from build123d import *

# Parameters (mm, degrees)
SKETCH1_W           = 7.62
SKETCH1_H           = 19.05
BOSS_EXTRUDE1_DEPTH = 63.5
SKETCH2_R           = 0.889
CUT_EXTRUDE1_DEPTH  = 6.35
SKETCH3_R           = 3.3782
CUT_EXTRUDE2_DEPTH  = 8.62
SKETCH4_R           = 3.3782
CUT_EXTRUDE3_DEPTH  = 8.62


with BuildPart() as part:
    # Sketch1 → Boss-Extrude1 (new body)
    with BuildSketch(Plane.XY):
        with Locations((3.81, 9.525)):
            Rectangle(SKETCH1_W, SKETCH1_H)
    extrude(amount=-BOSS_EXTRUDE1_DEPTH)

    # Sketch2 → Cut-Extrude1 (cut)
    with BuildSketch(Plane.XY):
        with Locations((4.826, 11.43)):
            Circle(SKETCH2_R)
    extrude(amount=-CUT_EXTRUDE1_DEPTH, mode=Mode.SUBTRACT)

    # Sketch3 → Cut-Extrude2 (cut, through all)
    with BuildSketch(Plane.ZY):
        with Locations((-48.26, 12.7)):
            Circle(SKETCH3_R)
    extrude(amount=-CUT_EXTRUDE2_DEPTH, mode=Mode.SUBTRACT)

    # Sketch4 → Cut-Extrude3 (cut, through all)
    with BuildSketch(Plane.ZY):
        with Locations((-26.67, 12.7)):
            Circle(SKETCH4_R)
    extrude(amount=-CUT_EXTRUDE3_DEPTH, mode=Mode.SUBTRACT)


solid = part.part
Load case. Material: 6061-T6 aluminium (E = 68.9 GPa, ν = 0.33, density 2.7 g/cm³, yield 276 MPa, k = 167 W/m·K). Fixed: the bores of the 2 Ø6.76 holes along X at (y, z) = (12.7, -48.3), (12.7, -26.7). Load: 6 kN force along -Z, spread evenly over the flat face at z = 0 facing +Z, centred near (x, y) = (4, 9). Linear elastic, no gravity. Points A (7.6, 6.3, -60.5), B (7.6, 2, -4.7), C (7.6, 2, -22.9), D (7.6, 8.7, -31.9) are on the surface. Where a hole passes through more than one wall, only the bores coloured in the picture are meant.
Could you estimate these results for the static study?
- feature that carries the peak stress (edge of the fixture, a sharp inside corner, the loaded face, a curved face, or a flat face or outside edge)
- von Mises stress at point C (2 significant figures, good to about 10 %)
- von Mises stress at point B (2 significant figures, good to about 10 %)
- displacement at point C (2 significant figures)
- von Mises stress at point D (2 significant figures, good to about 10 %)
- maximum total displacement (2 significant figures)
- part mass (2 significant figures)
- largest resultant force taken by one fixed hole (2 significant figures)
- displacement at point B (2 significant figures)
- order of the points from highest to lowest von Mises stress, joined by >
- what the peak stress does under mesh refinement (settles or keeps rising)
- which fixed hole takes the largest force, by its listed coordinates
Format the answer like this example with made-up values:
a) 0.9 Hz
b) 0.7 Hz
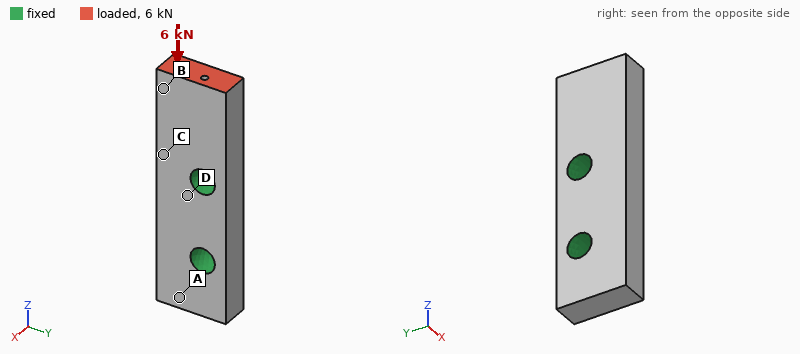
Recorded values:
a) edge of the fixture
b) 33 MPa
c) 42 MPa
d) 8.2 µm
e) 17 MPa
f) 26 µm
g) 23 g
h) 5.2 kN
i) 21 µm
j) B > C > D > A
k) keeps rising
l) (12.7, -26.7)
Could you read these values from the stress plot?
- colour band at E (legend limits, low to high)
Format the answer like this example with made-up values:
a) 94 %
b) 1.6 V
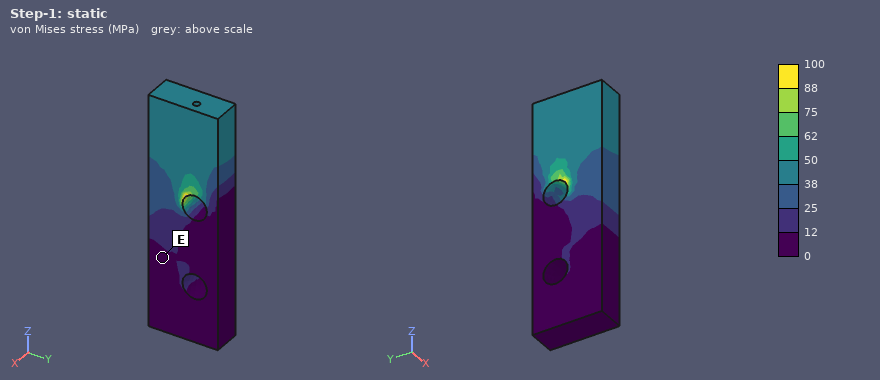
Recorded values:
a) 0 to 12 MPa
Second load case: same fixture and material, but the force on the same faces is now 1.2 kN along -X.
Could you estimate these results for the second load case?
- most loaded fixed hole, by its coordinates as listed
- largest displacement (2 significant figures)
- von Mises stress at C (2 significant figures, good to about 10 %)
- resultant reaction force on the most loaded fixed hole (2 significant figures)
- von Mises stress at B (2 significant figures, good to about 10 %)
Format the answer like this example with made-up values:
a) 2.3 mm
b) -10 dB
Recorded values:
a) (12.7, -26.7)
b) 0.15 mm
c) 90 MPa
d) 1.4 kN
e) 31 MPa
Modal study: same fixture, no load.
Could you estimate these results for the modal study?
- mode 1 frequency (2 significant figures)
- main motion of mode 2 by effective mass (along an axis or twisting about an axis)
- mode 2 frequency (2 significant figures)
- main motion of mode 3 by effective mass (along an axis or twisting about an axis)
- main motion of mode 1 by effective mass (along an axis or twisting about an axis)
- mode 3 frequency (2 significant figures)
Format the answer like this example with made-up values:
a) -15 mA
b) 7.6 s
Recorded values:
a) 9100 Hz
b) along Y
c) 14 kHz
d) twisting about Z
e) along X
f) 20 kHz
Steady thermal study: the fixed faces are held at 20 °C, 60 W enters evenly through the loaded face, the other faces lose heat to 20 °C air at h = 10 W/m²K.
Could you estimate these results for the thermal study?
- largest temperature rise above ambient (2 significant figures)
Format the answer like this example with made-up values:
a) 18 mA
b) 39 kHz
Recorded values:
a) 64 K
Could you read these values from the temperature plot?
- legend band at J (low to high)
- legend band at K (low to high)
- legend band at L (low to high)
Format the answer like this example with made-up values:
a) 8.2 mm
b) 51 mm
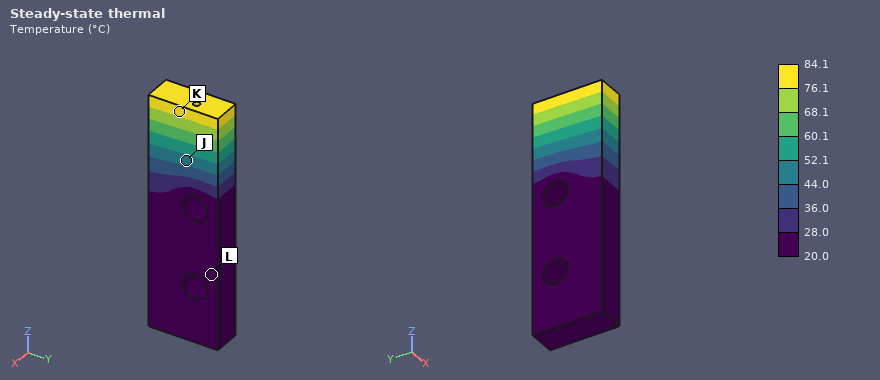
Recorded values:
a) 44.0 to 52.1 °C
b) 76.1 to 84.1 °C
c) 20.0 to 28.0 °C
